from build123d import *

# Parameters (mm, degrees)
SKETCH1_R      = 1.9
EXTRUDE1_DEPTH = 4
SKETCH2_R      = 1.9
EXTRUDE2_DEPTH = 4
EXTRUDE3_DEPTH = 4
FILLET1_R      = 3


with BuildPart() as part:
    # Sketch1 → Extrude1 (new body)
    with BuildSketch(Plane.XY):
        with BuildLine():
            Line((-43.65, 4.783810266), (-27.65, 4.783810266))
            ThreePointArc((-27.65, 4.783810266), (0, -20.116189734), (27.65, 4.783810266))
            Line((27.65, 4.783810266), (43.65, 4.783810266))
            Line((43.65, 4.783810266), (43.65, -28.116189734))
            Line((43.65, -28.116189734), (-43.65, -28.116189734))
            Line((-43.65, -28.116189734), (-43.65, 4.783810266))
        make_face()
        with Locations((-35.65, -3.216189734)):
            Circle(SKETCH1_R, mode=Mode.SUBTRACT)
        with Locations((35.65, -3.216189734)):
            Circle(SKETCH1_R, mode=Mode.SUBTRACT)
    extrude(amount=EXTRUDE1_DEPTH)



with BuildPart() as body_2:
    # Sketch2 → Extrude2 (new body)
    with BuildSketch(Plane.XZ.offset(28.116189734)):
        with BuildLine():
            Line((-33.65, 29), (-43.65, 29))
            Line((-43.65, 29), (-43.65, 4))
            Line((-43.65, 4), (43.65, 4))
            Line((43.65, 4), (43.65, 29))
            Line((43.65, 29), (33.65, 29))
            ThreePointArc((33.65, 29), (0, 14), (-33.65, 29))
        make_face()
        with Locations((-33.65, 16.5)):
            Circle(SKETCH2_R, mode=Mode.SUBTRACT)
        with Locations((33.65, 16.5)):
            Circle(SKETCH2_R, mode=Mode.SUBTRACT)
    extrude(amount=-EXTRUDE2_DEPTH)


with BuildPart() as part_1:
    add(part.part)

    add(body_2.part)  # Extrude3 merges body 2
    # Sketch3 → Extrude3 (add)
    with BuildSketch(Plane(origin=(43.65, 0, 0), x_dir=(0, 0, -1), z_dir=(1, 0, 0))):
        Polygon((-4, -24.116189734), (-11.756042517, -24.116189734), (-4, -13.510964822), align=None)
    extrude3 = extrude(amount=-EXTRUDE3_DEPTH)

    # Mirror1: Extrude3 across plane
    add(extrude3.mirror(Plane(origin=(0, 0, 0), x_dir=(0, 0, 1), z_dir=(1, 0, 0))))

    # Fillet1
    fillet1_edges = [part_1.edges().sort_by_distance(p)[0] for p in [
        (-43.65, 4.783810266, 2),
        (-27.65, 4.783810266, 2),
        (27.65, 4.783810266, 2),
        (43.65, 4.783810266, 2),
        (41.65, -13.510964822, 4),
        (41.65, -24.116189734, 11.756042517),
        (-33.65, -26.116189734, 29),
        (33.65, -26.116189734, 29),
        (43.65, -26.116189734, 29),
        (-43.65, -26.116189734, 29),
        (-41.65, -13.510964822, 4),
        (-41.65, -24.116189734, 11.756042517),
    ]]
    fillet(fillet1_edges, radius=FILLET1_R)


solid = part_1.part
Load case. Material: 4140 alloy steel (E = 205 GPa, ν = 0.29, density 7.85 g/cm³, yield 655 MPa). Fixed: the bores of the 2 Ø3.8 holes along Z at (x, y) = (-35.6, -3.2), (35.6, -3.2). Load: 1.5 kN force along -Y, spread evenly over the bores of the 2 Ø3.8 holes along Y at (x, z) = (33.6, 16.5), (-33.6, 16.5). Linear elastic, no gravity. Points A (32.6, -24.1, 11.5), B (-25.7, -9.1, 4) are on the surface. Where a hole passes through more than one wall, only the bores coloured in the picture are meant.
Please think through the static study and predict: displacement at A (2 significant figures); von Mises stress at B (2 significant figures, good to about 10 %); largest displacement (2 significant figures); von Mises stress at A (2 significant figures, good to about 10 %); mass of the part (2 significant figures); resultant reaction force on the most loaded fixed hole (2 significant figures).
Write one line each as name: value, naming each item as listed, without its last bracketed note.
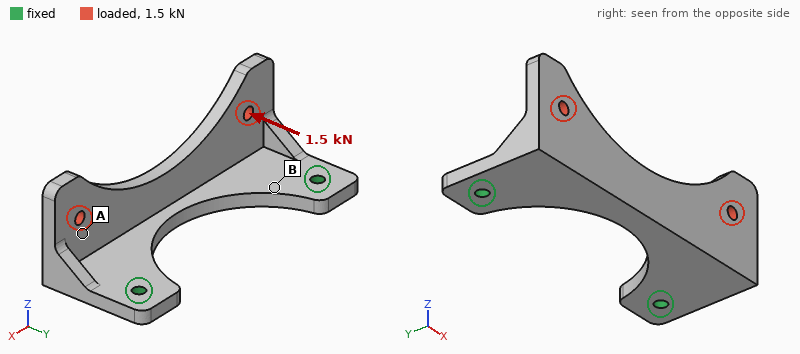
displacement at A: 0.13 mm
von Mises stress at B: 170 MPa
largest displacement: 0.28 mm
von Mises stress at A: 57 MPa
mass of the part: 100 g
resultant reaction force on the most loaded fixed hole: 750 N
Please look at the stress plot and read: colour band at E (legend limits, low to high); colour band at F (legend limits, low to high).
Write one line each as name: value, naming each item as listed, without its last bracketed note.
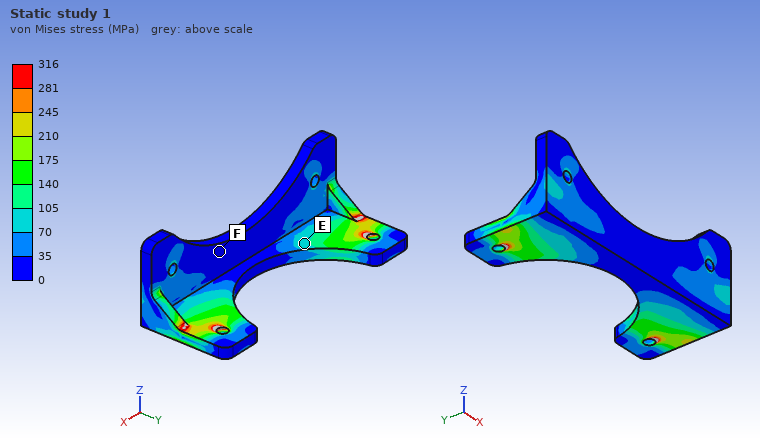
colour band at E: 70 to 105 MPa
colour band at F: 0 to 35 MPa
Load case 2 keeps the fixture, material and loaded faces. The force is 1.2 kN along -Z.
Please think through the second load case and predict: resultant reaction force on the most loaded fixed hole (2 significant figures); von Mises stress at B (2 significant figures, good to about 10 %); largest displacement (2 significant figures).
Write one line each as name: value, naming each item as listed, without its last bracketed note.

resultant reaction force on the most loaded fixed hole: 600 N
von Mises stress at B: 140 MPa
largest displacement: 0.21 mm
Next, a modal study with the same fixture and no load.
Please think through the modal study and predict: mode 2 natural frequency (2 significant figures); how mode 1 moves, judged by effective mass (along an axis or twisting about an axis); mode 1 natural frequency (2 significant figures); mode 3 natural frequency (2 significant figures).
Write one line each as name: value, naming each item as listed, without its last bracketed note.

mode 2 natural frequency: 2600 Hz
how mode 1 moves, judged by effective mass: along Z
mode 1 natural frequency: 1700 Hz
mode 3 natural frequency: 5700 Hz
